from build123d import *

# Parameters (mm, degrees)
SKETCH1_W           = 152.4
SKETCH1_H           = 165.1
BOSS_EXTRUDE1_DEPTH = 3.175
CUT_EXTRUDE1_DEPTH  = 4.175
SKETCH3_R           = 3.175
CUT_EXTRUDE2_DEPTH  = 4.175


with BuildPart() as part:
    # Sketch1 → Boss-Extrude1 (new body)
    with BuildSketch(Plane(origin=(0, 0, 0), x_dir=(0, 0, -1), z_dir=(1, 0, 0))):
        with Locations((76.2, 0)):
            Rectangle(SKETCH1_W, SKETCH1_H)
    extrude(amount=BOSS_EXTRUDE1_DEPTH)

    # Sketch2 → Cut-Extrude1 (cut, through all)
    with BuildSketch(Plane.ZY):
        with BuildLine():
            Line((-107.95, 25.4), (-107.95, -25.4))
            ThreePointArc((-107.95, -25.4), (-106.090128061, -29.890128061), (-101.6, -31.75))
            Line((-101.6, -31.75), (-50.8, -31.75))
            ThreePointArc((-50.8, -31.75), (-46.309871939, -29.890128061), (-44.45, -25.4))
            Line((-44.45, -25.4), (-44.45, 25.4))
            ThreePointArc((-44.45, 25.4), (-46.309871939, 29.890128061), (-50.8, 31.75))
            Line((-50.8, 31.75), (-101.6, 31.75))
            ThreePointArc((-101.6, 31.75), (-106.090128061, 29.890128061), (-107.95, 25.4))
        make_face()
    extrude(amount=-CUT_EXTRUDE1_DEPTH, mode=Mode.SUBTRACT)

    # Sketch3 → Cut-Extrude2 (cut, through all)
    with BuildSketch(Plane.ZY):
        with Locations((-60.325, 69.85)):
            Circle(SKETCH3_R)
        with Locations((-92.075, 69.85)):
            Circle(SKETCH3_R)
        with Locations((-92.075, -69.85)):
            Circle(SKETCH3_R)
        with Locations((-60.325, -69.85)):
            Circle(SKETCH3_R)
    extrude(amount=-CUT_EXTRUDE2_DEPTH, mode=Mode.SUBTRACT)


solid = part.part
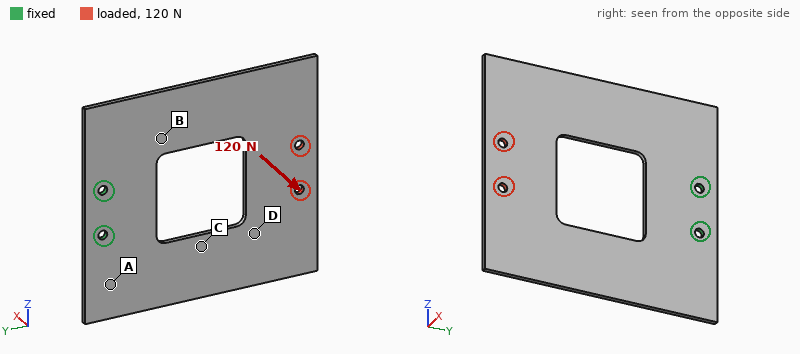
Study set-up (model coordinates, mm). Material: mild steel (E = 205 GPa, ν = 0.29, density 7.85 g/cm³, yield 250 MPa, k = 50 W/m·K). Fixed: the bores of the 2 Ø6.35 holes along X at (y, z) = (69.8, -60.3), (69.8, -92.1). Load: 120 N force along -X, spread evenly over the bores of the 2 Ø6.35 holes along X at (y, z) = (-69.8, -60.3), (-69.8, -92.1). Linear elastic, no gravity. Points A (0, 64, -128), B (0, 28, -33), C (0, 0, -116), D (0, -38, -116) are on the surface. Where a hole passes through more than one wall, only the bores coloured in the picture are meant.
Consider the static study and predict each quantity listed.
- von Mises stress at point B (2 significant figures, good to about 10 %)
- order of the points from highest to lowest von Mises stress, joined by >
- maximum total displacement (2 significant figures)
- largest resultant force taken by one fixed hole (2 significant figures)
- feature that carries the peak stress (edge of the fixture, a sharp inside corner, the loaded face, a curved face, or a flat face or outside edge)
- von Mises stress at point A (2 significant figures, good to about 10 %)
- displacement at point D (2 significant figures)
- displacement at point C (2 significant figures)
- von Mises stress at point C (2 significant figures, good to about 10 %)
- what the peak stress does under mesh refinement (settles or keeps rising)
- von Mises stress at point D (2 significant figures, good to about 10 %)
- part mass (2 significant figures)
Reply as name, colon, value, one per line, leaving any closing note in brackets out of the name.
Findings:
von Mises stress at point B: 87 MPa
order of the points from highest to lowest von Mises stress, joined by >: B > C > A > D
maximum total displacement: 2.6 mm
largest resultant force taken by one fixed hole: 60 N
feature that carries the peak stress: edge of the fixture
von Mises stress at point A: 45 MPa
displacement at point D: 1.5 mm
displacement at point C: 0.70 mm
von Mises stress at point C: 61 MPa
what the peak stress does under mesh refinement: keeps rising
von Mises stress at point D: 26 MPa
part mass: 520 g
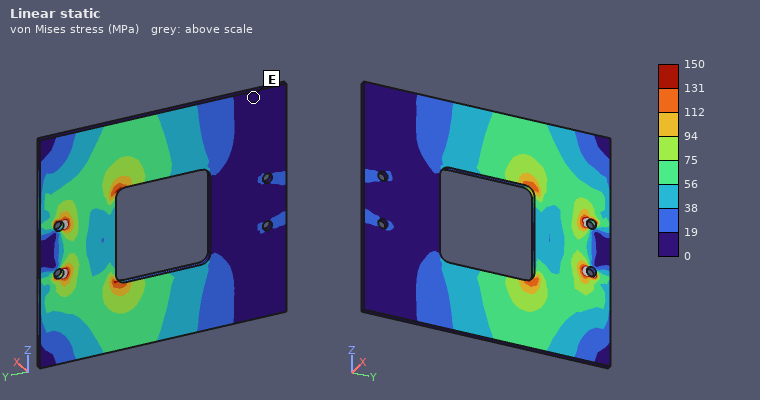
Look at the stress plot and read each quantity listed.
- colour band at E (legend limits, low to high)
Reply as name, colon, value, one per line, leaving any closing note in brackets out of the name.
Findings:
colour band at E: 0 to 19 MPa
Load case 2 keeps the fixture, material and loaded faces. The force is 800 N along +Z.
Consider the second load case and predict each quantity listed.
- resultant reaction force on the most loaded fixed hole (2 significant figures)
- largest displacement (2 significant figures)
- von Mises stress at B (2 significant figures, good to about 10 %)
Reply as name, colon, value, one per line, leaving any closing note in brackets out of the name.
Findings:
resultant reaction force on the most loaded fixed hole: 3.0 kN
largest displacement: 82 µm
von Mises stress at B: 12 MPa
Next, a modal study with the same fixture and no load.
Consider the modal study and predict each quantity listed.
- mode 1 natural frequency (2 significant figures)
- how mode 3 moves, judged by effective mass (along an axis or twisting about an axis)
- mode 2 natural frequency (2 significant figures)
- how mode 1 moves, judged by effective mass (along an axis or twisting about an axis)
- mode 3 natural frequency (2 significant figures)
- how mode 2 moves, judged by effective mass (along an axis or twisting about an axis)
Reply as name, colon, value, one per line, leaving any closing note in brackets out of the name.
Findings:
mode 1 natural frequency: 90 Hz
how mode 3 moves, judged by effective mass: along X
mode 2 natural frequency: 190 Hz
how mode 1 moves, judged by effective mass: along X
mode 3 natural frequency: 480 Hz
how mode 2 moves, judged by effective mass: twisting about Y
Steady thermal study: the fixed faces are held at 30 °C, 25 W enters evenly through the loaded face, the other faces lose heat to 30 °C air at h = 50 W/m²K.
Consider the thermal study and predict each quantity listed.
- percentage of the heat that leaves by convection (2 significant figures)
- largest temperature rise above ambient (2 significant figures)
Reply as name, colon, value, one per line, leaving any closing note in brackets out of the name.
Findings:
percentage of the heat that leaves by convection: 99 %
largest temperature rise above ambient: 64 K
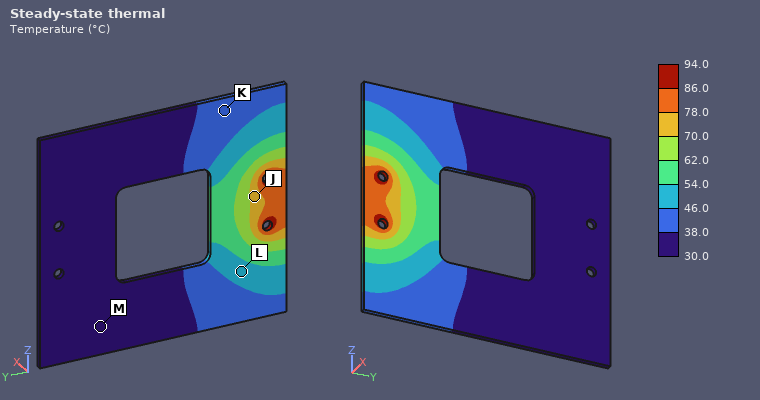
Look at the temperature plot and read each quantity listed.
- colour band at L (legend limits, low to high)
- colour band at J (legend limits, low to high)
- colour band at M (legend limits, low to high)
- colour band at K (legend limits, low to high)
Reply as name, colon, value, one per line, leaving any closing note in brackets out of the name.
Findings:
colour band at L: 46.0 to 54.0 °C
colour band at J: 70.0 to 78.0 °C
colour band at M: 30.0 to 38.0 °C
colour band at K: 38.0 to 46.0 °C
